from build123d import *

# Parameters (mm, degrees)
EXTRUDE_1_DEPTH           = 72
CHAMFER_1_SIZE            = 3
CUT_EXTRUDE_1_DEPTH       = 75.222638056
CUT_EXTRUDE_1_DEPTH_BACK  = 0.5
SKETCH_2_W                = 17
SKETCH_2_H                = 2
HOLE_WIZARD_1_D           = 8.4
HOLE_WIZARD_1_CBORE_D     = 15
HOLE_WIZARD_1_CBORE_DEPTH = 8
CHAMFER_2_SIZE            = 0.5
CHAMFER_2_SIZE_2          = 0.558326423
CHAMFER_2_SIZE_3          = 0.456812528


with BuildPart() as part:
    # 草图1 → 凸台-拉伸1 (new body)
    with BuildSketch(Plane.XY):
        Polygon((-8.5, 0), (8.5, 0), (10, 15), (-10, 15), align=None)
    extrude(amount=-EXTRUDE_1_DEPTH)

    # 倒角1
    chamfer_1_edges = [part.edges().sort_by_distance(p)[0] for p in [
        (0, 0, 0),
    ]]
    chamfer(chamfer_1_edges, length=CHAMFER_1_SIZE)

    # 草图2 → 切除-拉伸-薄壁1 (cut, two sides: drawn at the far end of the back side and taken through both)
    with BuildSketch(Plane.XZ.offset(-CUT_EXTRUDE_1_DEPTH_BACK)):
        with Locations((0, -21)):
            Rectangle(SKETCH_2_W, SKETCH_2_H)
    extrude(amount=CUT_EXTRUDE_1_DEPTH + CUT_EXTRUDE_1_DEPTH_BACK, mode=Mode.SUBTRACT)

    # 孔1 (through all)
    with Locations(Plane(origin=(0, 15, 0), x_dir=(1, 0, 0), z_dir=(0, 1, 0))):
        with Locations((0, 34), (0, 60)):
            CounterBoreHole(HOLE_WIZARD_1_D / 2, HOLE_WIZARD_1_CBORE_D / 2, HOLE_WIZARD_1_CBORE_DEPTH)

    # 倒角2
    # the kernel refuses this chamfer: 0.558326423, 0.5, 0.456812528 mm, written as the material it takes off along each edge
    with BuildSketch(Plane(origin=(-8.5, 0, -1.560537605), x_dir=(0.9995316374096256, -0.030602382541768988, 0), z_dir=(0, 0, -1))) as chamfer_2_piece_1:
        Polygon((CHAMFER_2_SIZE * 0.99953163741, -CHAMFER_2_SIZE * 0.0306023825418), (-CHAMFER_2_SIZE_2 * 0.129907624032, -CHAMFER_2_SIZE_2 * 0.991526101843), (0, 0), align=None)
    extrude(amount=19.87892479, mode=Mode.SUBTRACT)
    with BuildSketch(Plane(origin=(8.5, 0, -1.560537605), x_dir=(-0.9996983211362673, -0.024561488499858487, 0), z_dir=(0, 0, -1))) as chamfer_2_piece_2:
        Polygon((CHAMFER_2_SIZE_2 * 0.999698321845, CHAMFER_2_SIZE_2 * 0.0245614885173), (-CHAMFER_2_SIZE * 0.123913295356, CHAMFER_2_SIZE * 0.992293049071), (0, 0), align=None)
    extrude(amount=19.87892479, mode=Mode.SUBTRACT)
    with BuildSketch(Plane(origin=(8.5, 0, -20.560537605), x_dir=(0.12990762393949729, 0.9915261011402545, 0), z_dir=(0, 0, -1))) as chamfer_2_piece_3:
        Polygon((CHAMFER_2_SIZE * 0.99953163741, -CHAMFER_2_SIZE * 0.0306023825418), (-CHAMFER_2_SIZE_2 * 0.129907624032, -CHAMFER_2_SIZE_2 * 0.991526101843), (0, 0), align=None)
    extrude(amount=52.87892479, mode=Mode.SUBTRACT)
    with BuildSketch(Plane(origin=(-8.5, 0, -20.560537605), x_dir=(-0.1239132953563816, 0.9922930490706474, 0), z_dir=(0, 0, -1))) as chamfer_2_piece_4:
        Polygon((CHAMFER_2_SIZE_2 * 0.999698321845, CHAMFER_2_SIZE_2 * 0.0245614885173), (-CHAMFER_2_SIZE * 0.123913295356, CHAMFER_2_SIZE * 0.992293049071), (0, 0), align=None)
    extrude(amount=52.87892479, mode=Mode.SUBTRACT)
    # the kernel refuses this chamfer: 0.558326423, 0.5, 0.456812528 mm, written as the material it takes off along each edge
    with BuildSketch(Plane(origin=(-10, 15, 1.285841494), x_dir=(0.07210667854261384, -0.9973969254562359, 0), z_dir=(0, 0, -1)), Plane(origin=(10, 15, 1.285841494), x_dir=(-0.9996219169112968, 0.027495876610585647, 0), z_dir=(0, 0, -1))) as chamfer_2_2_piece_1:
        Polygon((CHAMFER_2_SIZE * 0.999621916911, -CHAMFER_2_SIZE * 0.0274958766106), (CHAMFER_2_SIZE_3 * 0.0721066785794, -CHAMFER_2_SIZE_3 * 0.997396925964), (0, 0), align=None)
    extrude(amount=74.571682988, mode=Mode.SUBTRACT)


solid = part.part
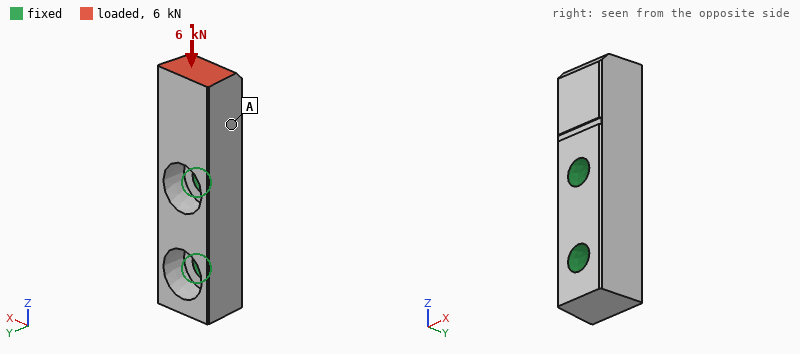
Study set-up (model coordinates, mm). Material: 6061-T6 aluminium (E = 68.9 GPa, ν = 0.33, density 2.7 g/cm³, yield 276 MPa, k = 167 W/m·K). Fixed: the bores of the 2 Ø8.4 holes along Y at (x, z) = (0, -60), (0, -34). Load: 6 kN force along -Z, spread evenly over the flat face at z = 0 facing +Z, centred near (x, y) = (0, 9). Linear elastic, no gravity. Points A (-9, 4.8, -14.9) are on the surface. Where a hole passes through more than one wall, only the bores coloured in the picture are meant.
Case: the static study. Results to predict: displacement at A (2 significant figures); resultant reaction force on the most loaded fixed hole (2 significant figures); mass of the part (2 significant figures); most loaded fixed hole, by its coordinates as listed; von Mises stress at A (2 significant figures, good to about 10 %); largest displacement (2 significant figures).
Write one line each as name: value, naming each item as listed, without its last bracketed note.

displacement at A: 30 µm
resultant reaction force on the most loaded fixed hole: 4.8 kN
mass of the part: 44 g
most loaded fixed hole, by its coordinates as listed: (0, -34)
von Mises stress at A: 19 MPa
largest displacement: 75 µm
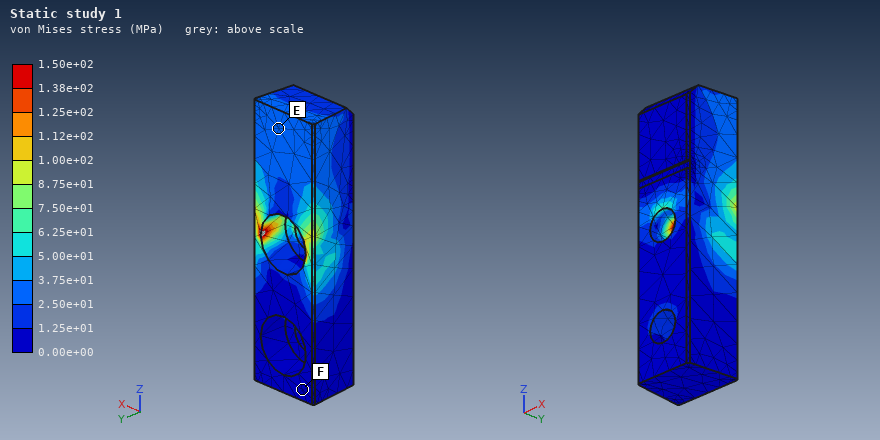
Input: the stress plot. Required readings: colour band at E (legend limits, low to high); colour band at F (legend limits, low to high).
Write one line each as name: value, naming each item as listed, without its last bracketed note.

colour band at E: 2.50e+01 to 3.75e+01 MPa
colour band at F: 0.00e+00 to 1.25e+01 MPa
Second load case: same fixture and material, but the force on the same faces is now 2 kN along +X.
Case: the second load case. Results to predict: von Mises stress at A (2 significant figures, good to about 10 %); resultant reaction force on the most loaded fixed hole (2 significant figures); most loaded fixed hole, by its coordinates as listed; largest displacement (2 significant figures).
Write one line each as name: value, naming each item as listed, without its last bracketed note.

von Mises stress at A: 35 MPa
resultant reaction force on the most loaded fixed hole: 3.0 kN
most loaded fixed hole, by its coordinates as listed: (0, -34)
largest displacement: 0.10 mm
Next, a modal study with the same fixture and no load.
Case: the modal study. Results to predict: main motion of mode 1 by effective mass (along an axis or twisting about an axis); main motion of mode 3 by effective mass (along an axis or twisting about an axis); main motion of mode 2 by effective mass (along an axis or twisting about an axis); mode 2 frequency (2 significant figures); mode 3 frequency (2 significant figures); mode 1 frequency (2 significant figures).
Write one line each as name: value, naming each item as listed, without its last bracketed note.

main motion of mode 1 by effective mass: along Y
main motion of mode 3 by effective mass: twisting about Z
main motion of mode 2 by effective mass: along X
mode 2 frequency: 8500 Hz
mode 3 frequency: 15 kHz
mode 1 frequency: 6600 Hz
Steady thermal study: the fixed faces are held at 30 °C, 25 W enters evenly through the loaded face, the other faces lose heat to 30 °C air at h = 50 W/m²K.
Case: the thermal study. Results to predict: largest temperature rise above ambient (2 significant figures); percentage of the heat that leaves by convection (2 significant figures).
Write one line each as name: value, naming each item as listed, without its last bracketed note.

largest temperature rise above ambient: 21 K
percentage of the heat that leaves by convection: 5.3 %
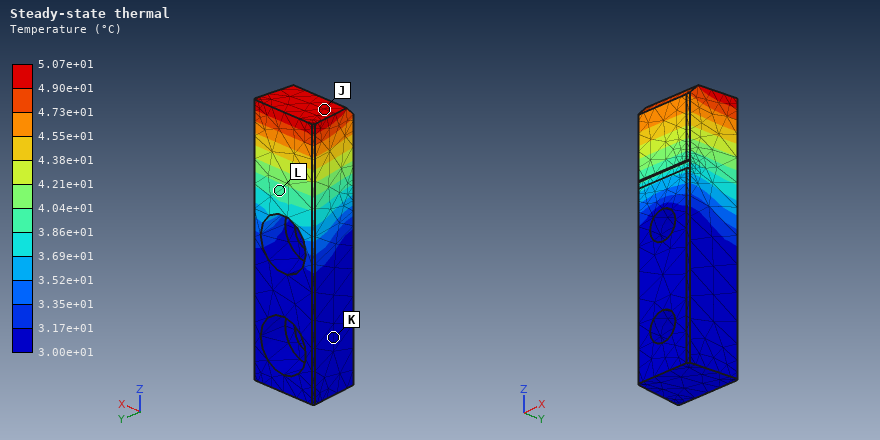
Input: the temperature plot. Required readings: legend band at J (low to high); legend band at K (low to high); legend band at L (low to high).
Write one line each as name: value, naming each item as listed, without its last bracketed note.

legend band at J: 4.90e+01 to 5.07e+01 °C
legend band at K: 3.00e+01 to 3.17e+01 °C
legend band at L: 3.86e+01 to 4.04e+01 °C
